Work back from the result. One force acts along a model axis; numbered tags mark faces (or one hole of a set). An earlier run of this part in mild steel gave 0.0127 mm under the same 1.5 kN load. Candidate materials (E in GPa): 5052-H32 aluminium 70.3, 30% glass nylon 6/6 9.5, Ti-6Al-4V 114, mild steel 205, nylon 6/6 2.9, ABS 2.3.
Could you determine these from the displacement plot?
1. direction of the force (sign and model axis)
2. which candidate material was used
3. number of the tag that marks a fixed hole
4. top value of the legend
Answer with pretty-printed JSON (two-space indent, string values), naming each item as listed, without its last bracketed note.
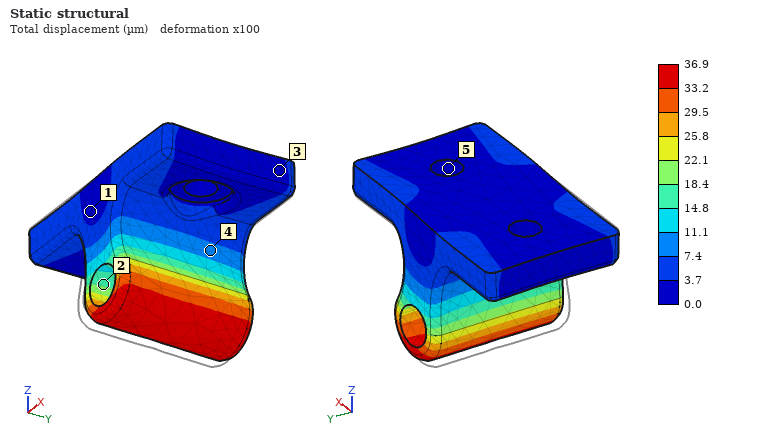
{
  "direction of the force": "+X",
  "which candidate material was used": "5052-H32 aluminium",
  "number of the tag that marks a fixed hole": "5",
  "top value of the legend": "36.9 µm"
}
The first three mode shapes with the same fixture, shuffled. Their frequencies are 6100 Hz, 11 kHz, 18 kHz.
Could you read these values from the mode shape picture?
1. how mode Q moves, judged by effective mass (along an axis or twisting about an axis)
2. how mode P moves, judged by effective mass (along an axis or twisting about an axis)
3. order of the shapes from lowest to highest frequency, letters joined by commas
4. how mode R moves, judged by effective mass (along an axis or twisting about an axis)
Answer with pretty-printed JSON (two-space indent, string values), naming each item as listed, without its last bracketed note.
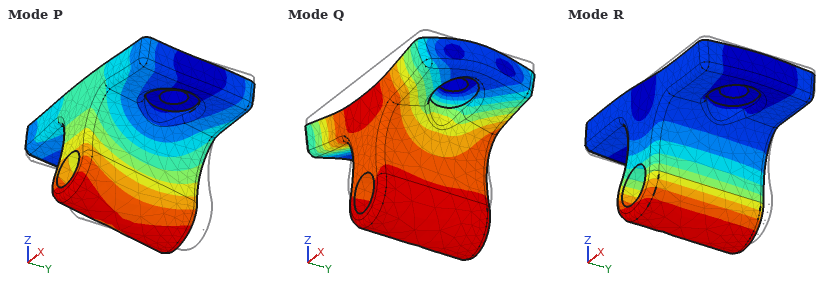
{
  "how mode Q moves, judged by effective mass": "along Z",
  "how mode P moves, judged by effective mass": "along Y",
  "order of the shapes from lowest to highest frequency, letters joined by commas": "P, R, Q",
  "how mode R moves, judged by effective mass": "along X"
}
